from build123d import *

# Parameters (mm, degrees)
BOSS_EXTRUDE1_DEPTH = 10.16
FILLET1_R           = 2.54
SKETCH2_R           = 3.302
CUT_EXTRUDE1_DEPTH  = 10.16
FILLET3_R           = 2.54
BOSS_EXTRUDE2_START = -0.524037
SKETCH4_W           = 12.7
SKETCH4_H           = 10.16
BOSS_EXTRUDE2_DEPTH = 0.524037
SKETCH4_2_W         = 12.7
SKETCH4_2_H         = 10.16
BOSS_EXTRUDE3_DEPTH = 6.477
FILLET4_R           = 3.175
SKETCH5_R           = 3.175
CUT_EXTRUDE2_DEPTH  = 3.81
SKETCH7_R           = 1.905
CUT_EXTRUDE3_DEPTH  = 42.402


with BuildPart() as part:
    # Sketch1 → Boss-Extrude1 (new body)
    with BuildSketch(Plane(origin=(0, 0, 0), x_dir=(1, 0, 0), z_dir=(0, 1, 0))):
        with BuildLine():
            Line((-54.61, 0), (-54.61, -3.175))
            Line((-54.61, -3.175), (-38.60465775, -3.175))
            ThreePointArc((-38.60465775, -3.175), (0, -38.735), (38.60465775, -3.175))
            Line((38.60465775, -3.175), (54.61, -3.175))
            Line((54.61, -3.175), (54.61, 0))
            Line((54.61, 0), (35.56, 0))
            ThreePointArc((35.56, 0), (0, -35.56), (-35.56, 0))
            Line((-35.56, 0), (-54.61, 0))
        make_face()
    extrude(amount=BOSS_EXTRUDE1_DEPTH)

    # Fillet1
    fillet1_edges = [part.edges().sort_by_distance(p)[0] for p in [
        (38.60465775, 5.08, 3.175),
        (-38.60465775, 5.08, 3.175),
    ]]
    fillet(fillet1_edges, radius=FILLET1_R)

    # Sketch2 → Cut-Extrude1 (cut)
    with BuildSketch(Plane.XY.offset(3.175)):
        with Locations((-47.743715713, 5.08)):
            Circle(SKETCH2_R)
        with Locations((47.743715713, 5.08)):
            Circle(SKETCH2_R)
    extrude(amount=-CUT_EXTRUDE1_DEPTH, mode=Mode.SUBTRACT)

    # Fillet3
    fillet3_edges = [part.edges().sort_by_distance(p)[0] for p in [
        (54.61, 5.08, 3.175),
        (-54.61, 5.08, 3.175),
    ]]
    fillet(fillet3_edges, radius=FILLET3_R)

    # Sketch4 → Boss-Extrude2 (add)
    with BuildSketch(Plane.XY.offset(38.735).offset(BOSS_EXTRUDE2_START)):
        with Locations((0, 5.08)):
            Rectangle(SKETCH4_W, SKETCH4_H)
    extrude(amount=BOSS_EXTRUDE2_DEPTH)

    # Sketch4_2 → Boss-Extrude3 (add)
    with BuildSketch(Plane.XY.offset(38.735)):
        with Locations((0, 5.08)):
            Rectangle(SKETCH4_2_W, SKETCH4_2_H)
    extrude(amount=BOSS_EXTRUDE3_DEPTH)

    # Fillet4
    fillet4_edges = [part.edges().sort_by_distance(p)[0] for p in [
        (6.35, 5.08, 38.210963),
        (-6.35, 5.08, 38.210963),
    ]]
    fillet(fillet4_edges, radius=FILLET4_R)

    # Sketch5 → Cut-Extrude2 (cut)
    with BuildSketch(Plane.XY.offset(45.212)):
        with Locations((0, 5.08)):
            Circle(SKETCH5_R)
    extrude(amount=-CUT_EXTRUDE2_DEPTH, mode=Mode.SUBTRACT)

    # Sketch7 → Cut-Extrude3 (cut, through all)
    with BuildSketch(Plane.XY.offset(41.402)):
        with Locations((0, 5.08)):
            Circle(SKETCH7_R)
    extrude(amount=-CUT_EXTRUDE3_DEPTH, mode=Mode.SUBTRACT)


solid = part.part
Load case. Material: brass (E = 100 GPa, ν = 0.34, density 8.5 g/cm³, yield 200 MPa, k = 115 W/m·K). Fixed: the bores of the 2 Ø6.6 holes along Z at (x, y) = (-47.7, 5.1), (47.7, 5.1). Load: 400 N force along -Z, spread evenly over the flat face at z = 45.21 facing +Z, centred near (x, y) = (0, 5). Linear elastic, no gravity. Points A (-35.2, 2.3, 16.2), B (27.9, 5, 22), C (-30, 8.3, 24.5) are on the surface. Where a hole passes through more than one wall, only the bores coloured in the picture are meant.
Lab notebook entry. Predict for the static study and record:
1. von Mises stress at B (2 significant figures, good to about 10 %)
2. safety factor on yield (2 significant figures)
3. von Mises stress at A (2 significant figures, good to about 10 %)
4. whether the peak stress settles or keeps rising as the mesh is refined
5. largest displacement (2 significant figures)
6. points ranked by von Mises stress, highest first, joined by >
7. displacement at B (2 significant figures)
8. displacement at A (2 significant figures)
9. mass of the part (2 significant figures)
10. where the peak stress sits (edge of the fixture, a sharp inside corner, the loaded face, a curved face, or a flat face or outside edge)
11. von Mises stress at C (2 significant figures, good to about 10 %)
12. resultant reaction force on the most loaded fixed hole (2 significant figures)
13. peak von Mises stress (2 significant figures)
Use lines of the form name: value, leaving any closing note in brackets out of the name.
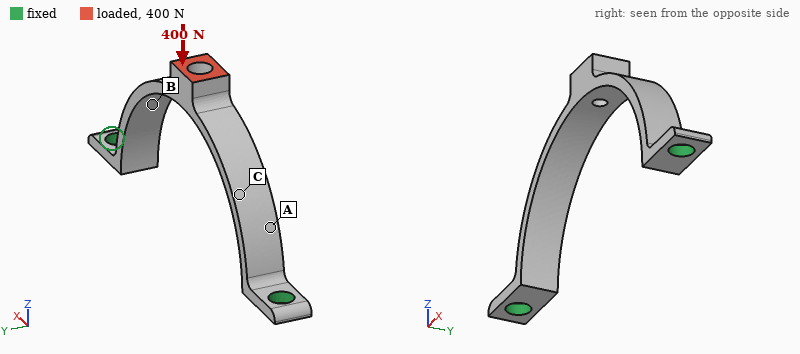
von Mises stress at B: 54 MPa
safety factor on yield: 2.3
von Mises stress at A: 16 MPa
whether the peak stress settles or keeps rising as the mesh is refined: settles
largest displacement: 50 µm
points ranked by von Mises stress, highest first, joined by >: B > C > A
displacement at B: 31 µm
displacement at A: 25 µm
mass of the part: 45 g
where the peak stress sits: a curved face
von Mises stress at C: 35 MPa
resultant reaction force on the most loaded fixed hole: 260 N
peak von Mises stress: 88 MPa
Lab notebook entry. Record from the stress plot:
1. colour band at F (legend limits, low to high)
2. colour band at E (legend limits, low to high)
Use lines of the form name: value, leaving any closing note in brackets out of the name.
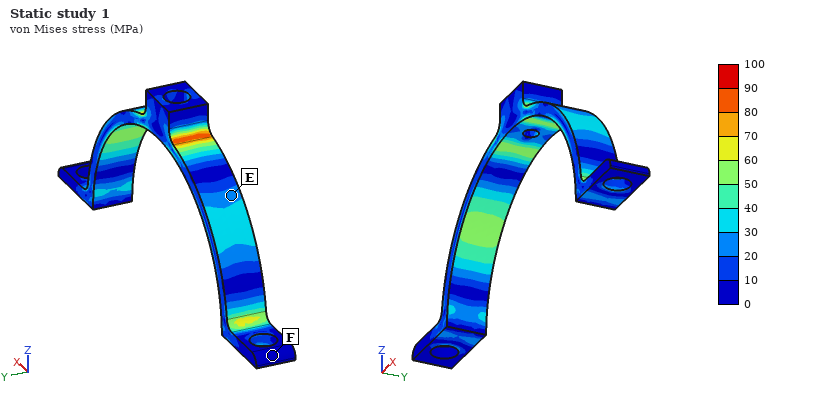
colour band at F: 0 to 10 MPa
colour band at E: 20 to 30 MPa
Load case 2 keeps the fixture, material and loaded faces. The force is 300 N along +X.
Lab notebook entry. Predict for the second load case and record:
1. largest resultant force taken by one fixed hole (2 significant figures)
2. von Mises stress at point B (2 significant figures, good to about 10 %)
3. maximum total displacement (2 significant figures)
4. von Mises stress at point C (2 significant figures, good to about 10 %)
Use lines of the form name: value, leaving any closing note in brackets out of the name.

largest resultant force taken by one fixed hole: 200 N
von Mises stress at point B: 47 MPa
maximum total displacement: 92 µm
von Mises stress at point C: 33 MPa
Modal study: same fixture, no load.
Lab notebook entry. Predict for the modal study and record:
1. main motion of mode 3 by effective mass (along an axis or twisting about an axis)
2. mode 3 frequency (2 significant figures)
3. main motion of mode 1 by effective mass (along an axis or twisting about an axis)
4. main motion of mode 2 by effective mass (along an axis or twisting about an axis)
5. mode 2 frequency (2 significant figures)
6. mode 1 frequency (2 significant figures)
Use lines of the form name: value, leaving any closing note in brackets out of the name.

main motion of mode 3 by effective mass: twisting about Z
mode 3 frequency: 3100 Hz
main motion of mode 1 by effective mass: along Y
main motion of mode 2 by effective mass: along X
mode 2 frequency: 1400 Hz
mode 1 frequency: 900 Hz
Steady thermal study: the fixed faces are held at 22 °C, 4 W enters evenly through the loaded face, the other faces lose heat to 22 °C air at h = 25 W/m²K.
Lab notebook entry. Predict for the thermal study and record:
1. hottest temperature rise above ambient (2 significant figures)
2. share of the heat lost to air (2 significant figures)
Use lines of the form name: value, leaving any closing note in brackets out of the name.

hottest temperature rise above ambient: 26 K
share of the heat lost to air: 31 %
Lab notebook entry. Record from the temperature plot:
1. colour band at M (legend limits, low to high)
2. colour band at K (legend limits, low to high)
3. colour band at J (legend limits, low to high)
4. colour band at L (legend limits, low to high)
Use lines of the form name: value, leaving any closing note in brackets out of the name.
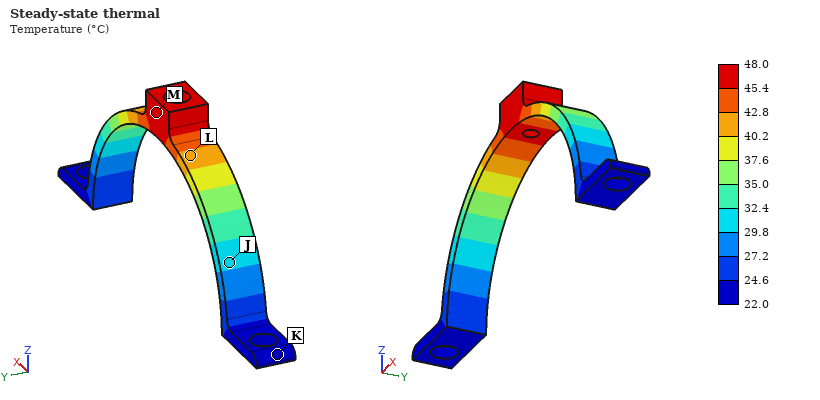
colour band at M: 45.4 to 48.0 °C
colour band at K: 22.0 to 24.6 °C
colour band at J: 29.8 to 32.4 °C
colour band at L: 40.2 to 42.8 °C
